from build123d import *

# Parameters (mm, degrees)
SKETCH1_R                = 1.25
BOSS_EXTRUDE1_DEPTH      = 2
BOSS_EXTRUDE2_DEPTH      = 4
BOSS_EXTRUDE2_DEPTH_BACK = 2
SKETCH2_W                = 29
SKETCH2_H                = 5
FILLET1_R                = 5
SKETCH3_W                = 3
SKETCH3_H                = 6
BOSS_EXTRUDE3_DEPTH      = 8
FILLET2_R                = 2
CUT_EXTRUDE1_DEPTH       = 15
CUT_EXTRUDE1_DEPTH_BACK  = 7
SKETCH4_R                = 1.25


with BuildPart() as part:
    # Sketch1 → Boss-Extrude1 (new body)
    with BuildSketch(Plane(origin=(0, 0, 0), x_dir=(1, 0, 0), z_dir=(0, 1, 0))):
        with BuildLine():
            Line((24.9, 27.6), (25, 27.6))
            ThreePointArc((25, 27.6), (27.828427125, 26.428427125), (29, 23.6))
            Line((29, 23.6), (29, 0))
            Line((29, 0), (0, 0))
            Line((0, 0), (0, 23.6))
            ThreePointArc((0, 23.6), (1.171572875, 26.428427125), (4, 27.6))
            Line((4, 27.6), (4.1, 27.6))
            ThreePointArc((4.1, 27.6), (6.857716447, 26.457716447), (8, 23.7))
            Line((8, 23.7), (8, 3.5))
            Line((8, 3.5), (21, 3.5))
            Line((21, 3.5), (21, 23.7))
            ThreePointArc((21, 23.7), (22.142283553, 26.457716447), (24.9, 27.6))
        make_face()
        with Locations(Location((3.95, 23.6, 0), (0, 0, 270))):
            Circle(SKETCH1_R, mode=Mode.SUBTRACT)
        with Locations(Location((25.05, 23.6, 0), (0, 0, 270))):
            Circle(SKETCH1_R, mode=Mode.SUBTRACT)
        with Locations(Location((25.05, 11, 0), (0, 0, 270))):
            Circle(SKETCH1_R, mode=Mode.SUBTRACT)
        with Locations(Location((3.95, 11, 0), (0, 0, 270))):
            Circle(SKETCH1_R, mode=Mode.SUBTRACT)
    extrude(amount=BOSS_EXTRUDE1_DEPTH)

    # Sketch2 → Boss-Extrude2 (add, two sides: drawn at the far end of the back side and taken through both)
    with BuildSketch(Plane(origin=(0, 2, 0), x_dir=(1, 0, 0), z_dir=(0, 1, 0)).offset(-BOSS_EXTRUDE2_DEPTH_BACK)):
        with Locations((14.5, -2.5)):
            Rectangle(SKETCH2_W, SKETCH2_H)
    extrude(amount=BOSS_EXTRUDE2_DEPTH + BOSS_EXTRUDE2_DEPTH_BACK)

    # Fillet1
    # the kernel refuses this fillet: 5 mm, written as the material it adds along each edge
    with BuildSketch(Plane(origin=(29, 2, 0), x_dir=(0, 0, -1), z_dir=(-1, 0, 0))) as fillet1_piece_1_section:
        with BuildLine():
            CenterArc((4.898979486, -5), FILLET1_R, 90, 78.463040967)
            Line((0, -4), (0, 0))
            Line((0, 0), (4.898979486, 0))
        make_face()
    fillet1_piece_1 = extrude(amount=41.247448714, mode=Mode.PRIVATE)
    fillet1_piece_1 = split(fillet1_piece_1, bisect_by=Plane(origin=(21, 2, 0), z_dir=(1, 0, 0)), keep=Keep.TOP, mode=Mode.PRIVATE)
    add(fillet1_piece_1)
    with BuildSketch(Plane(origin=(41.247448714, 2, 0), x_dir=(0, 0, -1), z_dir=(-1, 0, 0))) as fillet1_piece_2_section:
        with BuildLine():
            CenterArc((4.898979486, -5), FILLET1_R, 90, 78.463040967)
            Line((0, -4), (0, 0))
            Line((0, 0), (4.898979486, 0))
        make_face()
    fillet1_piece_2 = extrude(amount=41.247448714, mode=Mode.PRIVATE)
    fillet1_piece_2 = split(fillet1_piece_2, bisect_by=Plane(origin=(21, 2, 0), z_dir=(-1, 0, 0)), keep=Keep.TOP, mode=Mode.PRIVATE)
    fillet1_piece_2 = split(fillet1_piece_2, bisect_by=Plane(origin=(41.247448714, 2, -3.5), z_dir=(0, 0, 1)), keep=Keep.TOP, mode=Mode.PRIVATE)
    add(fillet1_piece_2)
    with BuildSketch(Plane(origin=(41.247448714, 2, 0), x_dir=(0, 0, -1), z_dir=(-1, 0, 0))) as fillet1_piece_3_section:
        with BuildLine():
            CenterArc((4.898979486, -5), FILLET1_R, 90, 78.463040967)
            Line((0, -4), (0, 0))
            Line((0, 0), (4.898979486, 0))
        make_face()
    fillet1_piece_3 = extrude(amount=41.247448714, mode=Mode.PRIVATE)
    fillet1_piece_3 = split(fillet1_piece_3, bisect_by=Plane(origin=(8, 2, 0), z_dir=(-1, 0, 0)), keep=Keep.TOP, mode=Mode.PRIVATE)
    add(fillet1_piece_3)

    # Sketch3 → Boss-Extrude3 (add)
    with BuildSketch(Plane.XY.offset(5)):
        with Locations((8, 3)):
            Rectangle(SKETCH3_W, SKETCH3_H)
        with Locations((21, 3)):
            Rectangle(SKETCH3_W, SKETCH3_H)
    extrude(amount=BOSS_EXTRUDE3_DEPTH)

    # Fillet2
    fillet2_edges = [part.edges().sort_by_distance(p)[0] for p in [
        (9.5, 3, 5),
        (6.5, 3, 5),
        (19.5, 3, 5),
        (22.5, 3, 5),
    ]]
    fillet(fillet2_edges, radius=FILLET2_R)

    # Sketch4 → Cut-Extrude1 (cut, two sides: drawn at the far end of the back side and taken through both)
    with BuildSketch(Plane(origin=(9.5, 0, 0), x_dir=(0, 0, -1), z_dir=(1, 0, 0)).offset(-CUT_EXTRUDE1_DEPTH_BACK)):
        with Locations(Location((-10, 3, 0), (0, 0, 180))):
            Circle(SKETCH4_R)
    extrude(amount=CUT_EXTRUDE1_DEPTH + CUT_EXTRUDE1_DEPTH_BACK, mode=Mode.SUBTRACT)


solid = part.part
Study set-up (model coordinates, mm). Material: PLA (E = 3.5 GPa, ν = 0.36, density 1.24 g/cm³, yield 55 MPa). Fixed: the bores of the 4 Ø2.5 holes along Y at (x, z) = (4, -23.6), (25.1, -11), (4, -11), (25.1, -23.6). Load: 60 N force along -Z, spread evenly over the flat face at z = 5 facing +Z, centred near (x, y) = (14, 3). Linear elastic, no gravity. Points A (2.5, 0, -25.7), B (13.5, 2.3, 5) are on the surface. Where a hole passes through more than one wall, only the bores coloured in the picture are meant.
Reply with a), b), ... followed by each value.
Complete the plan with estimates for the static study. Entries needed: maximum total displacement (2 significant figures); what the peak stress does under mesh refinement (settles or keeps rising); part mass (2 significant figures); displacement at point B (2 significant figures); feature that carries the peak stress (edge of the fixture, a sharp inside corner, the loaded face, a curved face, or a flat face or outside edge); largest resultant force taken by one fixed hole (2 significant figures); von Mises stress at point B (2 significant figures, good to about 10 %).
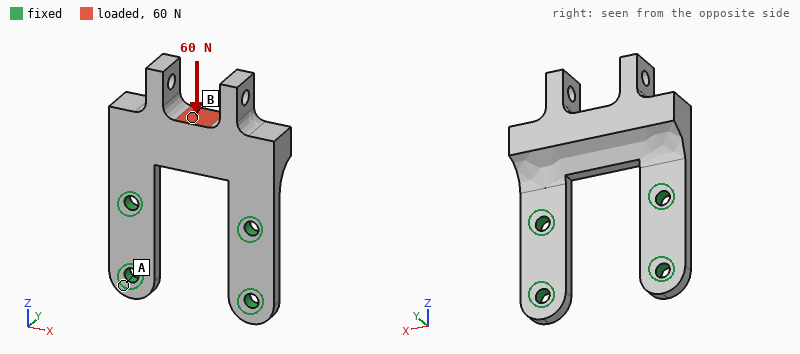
a) 0.50 mm
b) keeps rising
c) 2.7 g
d) 0.29 mm
e) edge of the fixture
f) 30 N
g) 3.5 MPa
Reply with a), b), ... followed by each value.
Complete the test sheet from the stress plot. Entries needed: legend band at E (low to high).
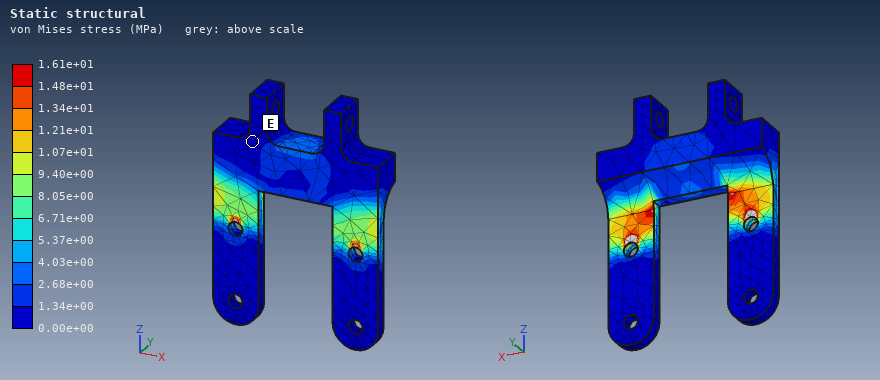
a) 0.00e+00 to 1.34e+00 MPa
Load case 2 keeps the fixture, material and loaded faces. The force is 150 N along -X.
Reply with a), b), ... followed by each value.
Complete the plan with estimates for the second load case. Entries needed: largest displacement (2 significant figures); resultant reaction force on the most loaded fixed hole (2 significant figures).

a) 0.12 mm
b) 120 N
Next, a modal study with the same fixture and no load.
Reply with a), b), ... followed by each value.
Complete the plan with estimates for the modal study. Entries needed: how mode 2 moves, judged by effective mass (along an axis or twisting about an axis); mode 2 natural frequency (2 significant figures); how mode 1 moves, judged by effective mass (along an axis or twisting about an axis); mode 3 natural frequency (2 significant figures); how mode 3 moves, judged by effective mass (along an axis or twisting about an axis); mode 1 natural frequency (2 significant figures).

a) twisting about Z
b) 3000 Hz
c) along Y
d) 4800 Hz
e) along X
f) 780 Hz
